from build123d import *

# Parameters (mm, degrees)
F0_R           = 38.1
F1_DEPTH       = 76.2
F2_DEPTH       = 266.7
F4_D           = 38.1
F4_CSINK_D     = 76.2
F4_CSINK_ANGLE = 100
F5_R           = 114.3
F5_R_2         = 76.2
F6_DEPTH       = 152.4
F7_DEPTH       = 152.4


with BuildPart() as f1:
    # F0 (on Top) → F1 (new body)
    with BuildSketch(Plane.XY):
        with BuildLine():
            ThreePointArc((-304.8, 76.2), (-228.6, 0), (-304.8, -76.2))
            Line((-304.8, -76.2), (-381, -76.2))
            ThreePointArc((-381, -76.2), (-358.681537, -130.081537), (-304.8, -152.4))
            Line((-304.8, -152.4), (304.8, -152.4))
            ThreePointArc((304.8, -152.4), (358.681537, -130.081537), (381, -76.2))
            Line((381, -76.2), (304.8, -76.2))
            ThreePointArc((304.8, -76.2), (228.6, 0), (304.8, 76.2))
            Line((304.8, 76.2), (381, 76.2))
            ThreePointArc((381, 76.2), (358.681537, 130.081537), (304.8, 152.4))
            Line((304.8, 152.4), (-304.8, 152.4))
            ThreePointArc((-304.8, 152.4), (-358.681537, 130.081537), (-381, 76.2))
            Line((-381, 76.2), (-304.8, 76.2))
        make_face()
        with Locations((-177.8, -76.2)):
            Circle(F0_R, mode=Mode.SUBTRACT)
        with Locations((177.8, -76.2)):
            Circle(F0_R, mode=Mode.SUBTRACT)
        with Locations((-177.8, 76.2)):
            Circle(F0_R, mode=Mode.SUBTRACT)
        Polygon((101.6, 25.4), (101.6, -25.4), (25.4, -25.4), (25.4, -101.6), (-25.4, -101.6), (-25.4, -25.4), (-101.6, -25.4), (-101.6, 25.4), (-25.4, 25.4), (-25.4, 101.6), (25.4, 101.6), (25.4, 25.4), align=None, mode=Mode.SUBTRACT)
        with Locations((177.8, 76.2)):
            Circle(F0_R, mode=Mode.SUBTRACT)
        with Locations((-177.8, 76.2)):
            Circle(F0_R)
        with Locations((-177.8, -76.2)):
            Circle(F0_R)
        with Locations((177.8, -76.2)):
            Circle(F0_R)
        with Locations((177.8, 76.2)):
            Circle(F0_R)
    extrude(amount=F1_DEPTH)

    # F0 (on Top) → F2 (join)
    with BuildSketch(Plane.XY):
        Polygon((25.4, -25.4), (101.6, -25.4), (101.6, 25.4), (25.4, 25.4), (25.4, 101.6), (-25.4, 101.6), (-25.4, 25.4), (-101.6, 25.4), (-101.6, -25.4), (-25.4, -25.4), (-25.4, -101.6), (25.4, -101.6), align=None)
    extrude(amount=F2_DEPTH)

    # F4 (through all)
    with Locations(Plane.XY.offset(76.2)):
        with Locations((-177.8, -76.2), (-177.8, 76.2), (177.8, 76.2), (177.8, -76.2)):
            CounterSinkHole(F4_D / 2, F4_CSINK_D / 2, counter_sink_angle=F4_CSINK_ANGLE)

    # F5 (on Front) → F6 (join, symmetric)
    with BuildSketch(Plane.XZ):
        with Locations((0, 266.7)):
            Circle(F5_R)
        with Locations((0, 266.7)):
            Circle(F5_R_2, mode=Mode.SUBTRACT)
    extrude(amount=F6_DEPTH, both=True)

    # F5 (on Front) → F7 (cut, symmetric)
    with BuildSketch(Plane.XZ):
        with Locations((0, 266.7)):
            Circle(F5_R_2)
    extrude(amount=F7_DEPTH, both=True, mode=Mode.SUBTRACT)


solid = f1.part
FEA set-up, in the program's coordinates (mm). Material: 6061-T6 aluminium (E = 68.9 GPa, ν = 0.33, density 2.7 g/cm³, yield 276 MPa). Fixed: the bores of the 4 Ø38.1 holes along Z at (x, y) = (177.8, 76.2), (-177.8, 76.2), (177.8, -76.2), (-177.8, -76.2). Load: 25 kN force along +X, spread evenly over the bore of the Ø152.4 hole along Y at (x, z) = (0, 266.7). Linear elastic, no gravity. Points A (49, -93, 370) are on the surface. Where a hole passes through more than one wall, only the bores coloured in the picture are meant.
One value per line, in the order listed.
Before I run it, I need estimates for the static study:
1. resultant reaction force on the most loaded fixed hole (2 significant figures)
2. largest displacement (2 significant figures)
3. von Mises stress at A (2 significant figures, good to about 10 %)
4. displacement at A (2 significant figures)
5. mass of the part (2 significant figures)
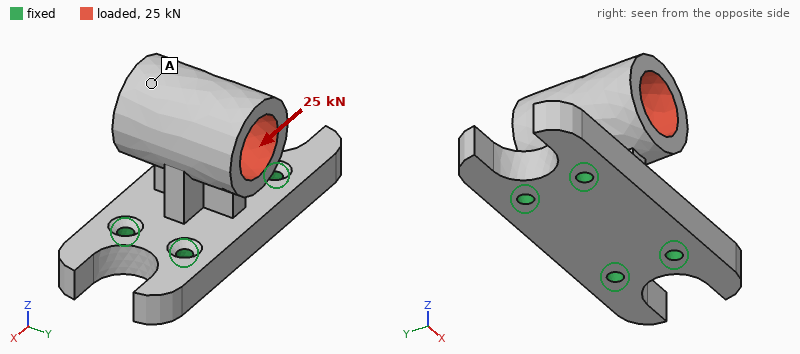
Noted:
12 kN
0.12 mm
1.7 MPa
0.12 mm
60 kg
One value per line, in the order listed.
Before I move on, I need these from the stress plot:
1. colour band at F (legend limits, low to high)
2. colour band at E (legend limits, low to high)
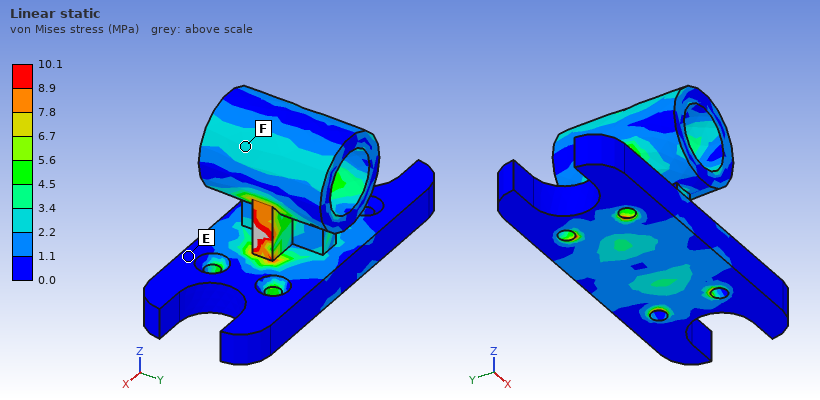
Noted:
2.2 to 3.4 MPa
0.0 to 1.1 MPa
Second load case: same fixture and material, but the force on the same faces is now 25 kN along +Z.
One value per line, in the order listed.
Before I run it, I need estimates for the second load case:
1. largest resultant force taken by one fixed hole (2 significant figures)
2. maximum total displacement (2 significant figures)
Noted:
6.7 kN
19 µm
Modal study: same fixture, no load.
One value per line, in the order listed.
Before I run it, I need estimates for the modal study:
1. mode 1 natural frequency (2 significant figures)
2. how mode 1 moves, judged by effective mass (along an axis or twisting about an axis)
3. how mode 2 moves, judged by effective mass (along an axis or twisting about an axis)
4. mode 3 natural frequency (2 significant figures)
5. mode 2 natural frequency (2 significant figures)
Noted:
500 Hz
along Y
along X
900 Hz
590 Hz
